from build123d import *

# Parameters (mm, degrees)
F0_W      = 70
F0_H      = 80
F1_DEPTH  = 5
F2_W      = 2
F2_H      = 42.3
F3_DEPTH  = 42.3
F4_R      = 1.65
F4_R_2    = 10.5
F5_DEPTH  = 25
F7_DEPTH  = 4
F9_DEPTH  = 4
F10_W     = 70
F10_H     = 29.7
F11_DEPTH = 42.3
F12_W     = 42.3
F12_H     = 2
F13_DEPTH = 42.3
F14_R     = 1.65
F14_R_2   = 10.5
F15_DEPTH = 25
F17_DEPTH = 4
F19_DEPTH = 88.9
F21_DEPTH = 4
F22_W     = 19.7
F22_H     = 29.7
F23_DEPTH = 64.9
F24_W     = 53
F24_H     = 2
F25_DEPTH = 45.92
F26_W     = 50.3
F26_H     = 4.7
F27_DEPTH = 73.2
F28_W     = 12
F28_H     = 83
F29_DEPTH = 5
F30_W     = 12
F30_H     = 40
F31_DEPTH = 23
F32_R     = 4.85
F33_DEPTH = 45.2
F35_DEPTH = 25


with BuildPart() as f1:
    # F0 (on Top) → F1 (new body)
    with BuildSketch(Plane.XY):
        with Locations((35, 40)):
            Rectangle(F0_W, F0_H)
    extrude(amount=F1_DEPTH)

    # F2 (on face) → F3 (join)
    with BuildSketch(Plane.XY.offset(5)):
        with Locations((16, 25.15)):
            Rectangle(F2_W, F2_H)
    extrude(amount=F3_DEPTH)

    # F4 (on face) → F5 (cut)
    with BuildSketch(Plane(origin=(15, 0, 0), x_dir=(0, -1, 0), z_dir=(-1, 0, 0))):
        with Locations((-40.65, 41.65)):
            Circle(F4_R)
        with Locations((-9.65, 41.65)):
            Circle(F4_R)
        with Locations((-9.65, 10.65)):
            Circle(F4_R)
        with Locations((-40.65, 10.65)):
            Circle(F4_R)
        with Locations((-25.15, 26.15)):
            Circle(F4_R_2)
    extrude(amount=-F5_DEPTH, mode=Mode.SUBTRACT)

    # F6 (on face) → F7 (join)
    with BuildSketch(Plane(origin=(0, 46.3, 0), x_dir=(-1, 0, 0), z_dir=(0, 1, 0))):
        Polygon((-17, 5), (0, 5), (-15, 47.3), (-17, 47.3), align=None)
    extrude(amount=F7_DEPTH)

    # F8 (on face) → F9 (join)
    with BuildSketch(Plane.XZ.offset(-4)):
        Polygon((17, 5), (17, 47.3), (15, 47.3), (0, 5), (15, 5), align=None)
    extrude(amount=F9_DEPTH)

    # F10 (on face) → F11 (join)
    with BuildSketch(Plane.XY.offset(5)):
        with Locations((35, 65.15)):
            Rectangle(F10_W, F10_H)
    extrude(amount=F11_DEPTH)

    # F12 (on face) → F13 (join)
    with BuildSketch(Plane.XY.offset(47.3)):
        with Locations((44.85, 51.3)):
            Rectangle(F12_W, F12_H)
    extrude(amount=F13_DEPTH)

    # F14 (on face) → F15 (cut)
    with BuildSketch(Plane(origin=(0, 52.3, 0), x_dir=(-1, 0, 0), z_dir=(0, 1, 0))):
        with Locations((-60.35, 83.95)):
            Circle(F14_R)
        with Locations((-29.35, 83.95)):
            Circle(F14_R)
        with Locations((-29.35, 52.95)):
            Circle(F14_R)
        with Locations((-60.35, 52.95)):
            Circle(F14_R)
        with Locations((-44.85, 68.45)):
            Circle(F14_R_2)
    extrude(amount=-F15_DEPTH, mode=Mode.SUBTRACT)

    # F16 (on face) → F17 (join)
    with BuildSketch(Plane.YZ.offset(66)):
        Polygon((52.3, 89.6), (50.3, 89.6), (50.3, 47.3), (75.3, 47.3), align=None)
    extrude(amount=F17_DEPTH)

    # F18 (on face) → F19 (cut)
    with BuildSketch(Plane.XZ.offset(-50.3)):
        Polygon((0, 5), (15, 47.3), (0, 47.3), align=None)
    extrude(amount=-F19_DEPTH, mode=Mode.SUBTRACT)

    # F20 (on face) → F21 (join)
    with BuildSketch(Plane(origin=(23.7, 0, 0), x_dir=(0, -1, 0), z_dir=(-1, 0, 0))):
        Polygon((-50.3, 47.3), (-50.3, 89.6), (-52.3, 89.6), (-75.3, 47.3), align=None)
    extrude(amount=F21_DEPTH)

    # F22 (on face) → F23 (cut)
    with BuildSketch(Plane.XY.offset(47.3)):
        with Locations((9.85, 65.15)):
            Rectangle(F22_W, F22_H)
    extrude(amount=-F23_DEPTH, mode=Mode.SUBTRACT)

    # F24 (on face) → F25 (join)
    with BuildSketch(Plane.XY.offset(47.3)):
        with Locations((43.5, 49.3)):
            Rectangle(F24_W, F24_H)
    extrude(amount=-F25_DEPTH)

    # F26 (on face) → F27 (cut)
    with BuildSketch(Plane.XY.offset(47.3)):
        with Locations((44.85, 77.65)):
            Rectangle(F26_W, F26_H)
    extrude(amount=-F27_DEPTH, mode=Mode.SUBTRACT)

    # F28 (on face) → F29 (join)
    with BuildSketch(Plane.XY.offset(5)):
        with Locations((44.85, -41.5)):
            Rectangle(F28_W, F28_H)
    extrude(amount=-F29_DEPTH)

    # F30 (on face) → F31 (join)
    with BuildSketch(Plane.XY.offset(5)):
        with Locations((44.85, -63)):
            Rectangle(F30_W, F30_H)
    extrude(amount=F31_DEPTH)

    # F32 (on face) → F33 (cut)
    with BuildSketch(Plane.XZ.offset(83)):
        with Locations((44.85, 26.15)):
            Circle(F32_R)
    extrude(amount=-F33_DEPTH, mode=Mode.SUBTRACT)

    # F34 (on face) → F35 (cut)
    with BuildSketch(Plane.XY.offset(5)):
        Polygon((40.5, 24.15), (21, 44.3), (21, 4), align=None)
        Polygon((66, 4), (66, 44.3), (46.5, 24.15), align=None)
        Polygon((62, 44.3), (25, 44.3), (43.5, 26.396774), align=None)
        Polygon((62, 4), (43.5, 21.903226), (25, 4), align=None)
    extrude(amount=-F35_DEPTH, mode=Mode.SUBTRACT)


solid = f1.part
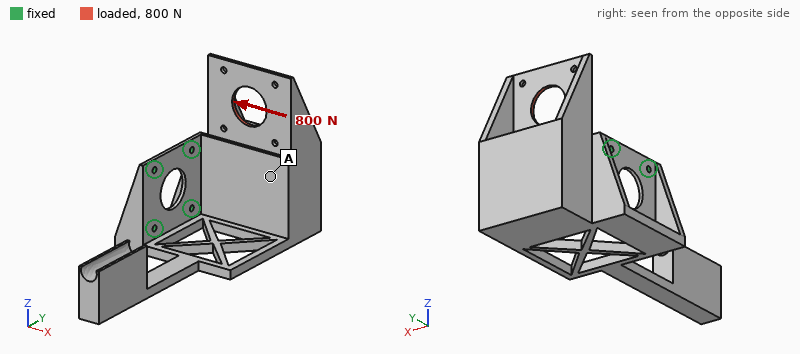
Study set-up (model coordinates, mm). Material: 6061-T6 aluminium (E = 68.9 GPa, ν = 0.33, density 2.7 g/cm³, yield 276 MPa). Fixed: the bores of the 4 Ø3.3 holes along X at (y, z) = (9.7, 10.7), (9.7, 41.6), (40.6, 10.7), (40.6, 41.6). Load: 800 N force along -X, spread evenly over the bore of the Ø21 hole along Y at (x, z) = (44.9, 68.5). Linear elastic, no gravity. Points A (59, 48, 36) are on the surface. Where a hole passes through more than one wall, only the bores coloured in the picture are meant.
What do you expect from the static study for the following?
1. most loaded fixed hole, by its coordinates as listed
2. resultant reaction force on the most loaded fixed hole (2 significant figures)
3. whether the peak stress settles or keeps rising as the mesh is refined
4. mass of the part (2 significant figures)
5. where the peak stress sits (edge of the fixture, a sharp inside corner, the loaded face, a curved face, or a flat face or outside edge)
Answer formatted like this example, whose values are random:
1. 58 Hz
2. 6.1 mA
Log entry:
1. (40.6, 41.6)
2. 1.4 kN
3. keeps rising
4. 270 g
5. edge of the fixture
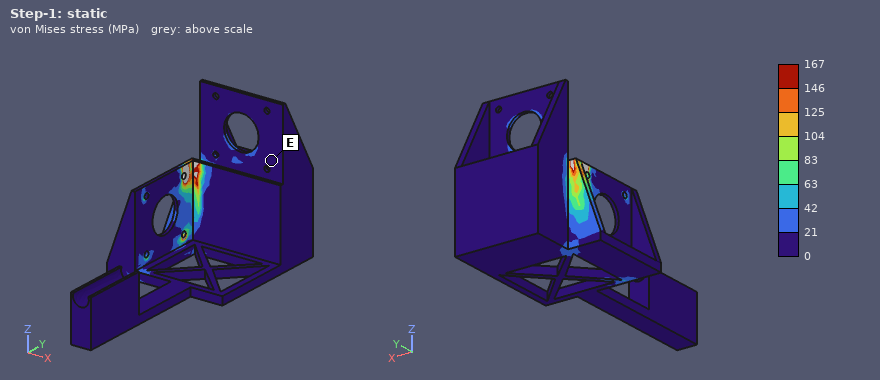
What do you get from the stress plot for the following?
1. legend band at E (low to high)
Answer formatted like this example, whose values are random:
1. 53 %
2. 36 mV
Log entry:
1. 0 to 21 MPa
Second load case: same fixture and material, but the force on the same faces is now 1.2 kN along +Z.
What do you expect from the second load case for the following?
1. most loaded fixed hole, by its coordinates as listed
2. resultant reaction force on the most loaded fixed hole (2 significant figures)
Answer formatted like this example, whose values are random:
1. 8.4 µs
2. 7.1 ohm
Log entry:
1. (40.6, 10.7)
2. 1.4 kN
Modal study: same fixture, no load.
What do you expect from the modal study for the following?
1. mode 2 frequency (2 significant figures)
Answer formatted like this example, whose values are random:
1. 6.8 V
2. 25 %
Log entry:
1. 340 Hz
